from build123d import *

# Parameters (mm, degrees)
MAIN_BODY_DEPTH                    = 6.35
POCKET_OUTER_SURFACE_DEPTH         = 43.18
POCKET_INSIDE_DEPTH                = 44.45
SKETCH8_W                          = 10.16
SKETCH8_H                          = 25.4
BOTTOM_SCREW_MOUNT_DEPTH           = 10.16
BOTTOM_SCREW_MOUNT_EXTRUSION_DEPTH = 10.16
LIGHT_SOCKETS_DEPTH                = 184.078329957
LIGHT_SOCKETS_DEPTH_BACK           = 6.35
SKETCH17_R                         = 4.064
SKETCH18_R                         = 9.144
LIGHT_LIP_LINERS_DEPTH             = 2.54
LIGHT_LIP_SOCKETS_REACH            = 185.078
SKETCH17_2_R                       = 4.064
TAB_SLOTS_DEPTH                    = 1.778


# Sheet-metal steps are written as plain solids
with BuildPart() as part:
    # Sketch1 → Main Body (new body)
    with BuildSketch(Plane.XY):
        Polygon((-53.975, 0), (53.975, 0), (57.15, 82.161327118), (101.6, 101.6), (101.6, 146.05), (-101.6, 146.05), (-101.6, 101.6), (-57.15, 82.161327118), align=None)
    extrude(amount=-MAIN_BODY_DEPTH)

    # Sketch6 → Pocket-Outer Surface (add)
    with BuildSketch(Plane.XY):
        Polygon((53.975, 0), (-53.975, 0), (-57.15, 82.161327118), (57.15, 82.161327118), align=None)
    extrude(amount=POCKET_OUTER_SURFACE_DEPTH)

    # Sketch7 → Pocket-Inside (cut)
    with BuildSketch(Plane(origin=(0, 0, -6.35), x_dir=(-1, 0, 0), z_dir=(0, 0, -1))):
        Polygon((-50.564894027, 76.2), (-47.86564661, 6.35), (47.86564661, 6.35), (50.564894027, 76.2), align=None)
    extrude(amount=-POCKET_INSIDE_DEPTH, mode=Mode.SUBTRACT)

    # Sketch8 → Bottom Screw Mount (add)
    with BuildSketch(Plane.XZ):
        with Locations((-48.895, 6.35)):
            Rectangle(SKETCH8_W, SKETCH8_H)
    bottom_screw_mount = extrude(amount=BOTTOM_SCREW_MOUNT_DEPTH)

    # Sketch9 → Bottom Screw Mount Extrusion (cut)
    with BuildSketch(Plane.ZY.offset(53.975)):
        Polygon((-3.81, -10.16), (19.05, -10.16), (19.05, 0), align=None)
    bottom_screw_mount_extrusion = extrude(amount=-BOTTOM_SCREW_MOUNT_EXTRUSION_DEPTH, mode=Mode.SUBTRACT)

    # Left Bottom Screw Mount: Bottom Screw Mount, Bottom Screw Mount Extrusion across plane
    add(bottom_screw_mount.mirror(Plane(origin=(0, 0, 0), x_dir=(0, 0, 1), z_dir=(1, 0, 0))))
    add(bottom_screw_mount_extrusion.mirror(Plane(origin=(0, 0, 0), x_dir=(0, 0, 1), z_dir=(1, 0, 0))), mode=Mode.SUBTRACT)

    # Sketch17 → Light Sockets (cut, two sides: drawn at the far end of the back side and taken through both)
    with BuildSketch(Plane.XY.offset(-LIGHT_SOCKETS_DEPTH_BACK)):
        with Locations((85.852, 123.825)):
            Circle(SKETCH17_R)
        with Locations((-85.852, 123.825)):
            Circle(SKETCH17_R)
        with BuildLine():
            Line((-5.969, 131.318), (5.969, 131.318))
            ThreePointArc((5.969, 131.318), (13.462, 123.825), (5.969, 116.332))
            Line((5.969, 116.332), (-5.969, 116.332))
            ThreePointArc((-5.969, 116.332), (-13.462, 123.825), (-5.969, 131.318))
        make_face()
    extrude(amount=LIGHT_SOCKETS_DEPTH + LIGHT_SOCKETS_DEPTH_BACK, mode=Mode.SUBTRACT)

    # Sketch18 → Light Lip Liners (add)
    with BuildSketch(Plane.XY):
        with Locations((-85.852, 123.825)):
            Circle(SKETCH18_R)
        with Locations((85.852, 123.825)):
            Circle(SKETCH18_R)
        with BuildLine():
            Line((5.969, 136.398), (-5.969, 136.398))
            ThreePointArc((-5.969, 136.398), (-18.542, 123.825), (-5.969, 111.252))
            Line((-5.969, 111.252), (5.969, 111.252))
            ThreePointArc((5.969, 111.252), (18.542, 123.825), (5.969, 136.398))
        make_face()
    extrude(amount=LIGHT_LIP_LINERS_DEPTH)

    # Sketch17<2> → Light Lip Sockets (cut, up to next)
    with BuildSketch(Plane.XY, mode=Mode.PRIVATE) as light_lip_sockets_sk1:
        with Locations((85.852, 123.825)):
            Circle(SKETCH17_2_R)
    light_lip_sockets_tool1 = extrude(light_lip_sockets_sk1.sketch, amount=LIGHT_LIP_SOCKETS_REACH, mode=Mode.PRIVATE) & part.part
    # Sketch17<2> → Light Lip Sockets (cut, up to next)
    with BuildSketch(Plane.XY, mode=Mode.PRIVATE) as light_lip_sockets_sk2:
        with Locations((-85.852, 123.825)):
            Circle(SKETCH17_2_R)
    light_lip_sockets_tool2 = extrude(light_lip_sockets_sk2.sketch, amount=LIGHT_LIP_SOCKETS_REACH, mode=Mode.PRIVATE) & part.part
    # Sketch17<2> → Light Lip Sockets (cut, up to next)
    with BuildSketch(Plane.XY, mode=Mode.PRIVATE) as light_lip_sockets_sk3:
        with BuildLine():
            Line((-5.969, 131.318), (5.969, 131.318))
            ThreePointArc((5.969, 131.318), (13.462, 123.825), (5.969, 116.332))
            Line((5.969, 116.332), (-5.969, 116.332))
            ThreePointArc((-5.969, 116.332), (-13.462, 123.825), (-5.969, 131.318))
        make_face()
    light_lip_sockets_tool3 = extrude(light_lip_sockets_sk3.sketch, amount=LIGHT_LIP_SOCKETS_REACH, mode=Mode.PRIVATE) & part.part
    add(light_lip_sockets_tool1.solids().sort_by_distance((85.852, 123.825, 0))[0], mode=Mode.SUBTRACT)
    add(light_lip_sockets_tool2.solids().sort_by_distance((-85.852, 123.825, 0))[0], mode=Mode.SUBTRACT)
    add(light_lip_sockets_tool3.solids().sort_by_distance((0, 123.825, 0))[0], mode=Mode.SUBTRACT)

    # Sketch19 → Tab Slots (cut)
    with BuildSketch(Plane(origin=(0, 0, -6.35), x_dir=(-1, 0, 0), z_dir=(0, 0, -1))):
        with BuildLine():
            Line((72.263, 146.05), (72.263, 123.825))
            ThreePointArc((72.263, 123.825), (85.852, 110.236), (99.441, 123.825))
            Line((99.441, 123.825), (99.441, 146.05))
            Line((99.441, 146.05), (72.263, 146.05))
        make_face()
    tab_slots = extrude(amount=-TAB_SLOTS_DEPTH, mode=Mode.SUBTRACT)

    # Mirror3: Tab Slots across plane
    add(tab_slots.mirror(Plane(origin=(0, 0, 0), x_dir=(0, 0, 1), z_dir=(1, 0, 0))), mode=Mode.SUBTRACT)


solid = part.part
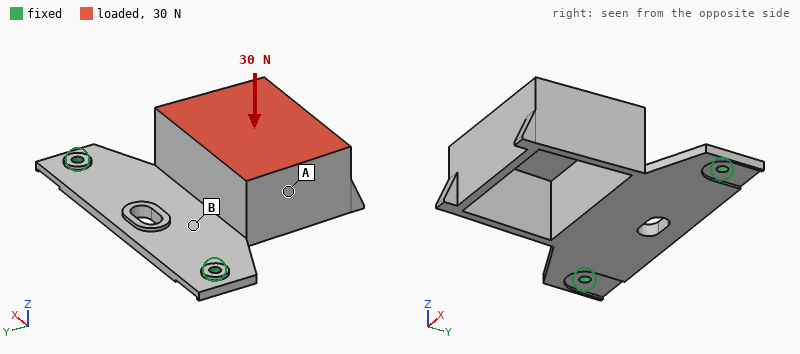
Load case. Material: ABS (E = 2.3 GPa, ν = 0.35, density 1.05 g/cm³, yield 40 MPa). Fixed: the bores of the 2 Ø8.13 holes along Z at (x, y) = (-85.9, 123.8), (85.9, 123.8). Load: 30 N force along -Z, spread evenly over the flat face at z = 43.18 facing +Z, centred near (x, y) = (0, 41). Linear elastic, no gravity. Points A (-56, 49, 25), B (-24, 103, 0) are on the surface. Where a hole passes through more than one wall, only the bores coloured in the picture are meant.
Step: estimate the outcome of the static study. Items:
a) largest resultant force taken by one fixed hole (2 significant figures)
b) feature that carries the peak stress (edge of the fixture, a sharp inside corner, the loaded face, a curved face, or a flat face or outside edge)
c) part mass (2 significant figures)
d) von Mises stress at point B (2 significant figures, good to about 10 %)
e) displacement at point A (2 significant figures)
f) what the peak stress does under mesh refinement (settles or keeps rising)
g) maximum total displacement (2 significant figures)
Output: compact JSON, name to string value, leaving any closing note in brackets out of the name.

{"largest resultant force taken by one fixed hole": "16 N", "feature that carries the peak stress": "edge of the fixture", "part mass": "230 g", "von Mises stress at point B": "1.1 MPa", "displacement at point A": "1.4 mm", "what the peak stress does under mesh refinement": "keeps rising", "maximum total displacement": "2.5 mm"}
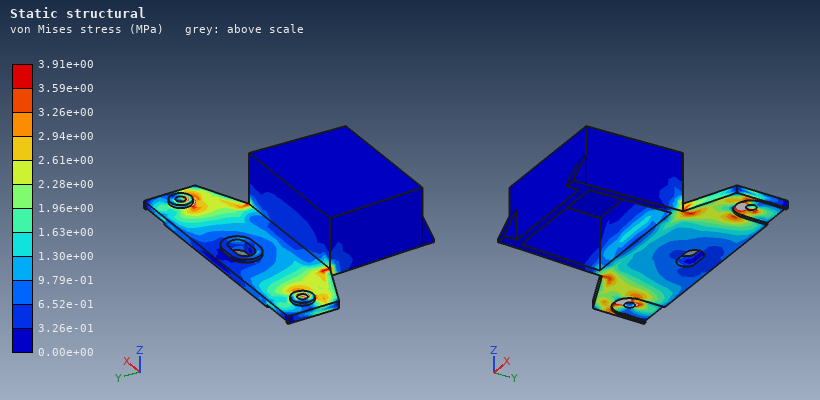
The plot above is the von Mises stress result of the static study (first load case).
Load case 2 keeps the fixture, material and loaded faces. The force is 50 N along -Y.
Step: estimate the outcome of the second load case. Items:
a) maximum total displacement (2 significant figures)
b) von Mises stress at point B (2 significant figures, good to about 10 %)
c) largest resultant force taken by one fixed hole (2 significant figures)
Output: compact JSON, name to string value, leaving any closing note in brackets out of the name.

{"maximum total displacement": "2.9 mm", "von Mises stress at point B": "1.7 MPa", "largest resultant force taken by one fixed hole": "26 N"}
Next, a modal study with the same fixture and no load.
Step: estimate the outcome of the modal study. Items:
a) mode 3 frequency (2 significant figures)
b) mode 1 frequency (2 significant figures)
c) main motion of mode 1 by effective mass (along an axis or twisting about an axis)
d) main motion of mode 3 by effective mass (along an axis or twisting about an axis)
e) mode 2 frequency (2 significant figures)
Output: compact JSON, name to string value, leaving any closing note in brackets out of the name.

{"mode 3 frequency": "250 Hz", "mode 1 frequency": "49 Hz", "main motion of mode 1 by effective mass": "along Z", "main motion of mode 3 by effective mass": "along X", "mode 2 frequency": "190 Hz"}
